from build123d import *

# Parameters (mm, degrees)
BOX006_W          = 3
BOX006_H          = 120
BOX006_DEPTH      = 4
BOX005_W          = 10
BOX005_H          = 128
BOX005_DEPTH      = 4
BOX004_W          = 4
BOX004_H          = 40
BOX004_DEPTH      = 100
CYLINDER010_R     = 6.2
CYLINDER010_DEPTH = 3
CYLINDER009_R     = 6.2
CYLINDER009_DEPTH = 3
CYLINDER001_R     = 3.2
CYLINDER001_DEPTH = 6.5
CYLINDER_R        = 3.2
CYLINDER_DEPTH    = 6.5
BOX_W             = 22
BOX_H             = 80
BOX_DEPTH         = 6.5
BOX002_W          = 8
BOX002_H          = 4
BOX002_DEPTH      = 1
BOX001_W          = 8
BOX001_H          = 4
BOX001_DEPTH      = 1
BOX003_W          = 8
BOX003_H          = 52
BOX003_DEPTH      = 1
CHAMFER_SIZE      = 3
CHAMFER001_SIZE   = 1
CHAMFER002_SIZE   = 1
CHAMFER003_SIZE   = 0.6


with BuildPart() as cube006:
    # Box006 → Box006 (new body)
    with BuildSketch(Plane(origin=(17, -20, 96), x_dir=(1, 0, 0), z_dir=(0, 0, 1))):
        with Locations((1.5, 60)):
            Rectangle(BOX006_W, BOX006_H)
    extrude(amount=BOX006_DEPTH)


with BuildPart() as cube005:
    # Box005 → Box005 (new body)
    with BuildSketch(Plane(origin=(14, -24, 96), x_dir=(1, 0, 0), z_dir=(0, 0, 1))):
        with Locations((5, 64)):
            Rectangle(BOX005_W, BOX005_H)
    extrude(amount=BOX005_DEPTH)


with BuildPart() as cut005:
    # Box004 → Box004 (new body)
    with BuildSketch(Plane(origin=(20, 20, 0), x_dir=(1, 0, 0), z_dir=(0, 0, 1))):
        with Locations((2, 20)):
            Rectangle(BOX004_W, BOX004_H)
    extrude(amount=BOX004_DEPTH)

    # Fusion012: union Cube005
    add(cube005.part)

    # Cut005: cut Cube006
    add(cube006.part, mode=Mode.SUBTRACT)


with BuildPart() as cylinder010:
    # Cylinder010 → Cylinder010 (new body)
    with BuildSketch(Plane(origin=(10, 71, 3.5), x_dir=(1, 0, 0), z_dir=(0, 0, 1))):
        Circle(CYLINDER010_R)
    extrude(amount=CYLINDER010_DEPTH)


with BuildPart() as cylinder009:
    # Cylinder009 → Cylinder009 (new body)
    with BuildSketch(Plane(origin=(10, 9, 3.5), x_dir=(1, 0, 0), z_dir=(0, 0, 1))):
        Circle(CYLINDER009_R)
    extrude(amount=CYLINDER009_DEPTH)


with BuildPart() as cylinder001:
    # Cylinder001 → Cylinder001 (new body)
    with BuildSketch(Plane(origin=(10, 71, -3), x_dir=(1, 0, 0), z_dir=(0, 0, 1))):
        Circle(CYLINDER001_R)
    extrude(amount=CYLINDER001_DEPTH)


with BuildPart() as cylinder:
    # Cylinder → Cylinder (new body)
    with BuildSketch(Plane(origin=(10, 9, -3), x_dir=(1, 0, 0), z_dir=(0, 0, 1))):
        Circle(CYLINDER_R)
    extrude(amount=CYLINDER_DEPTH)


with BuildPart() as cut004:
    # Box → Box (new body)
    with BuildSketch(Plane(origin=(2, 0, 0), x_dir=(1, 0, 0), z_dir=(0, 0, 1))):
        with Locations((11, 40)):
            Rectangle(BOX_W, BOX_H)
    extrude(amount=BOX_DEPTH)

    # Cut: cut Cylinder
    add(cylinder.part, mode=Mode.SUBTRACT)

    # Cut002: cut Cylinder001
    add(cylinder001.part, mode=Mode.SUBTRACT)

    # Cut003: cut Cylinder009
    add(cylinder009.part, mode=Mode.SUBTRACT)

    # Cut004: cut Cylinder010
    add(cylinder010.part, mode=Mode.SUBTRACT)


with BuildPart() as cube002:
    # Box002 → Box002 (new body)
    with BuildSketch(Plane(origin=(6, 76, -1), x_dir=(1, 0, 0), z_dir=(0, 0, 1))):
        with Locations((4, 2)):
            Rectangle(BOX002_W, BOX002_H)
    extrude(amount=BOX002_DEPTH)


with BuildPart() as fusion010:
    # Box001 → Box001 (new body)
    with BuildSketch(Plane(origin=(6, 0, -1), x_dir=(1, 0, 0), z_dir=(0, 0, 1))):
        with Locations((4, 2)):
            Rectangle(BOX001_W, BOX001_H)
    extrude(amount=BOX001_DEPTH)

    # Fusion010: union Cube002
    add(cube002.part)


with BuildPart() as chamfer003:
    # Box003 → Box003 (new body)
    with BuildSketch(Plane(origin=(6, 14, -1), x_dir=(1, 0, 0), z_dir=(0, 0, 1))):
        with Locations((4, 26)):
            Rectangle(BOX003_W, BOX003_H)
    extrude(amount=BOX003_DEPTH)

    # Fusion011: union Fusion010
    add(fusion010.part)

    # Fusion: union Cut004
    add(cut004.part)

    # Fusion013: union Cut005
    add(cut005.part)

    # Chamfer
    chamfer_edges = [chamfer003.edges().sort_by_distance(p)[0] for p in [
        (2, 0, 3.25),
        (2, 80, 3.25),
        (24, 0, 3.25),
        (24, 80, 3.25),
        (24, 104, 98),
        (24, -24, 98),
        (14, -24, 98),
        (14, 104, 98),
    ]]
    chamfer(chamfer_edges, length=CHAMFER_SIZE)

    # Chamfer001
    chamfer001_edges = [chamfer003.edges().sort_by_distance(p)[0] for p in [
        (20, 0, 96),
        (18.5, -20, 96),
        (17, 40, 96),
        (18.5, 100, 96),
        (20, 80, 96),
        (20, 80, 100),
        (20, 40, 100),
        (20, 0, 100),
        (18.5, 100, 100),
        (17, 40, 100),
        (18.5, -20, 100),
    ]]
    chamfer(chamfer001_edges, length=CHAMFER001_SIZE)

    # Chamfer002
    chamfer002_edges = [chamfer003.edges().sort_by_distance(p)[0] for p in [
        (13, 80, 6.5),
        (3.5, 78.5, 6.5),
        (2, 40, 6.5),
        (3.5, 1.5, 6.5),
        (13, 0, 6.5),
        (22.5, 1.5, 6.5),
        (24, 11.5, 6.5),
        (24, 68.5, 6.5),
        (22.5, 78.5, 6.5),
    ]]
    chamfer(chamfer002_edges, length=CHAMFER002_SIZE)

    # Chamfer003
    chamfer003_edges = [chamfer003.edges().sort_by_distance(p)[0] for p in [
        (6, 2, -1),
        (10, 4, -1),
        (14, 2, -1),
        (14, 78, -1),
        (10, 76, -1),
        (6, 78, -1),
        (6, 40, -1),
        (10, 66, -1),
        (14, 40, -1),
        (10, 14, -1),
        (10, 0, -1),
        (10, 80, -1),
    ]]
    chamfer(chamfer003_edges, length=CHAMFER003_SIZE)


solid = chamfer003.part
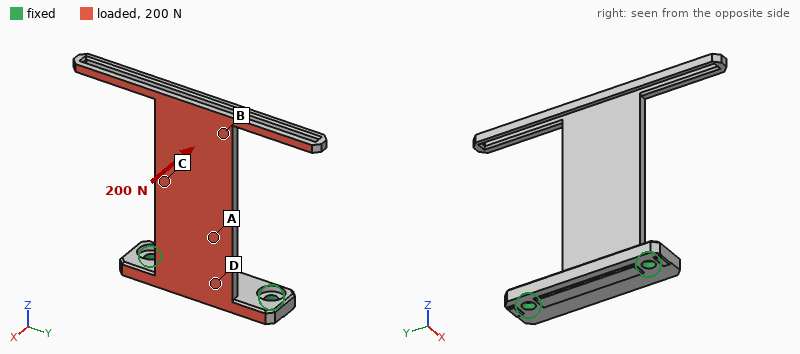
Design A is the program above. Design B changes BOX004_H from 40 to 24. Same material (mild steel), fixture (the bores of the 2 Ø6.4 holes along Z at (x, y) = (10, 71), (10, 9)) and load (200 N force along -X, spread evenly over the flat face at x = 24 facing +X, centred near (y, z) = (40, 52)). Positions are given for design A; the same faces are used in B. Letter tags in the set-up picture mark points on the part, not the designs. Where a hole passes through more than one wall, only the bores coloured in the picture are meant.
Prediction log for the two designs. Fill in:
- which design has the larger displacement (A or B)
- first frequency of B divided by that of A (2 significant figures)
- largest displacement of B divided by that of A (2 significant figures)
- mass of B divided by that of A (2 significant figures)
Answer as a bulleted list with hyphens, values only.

- B
- 0.88
- 1.7
- 0.80
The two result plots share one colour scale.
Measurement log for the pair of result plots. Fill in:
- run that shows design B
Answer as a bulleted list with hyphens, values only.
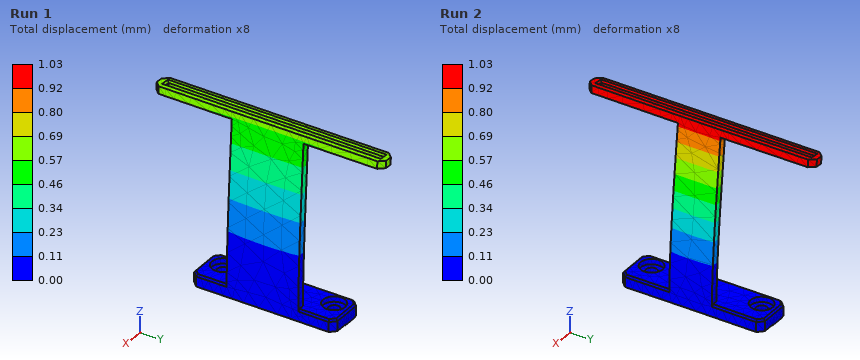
- Run 2
